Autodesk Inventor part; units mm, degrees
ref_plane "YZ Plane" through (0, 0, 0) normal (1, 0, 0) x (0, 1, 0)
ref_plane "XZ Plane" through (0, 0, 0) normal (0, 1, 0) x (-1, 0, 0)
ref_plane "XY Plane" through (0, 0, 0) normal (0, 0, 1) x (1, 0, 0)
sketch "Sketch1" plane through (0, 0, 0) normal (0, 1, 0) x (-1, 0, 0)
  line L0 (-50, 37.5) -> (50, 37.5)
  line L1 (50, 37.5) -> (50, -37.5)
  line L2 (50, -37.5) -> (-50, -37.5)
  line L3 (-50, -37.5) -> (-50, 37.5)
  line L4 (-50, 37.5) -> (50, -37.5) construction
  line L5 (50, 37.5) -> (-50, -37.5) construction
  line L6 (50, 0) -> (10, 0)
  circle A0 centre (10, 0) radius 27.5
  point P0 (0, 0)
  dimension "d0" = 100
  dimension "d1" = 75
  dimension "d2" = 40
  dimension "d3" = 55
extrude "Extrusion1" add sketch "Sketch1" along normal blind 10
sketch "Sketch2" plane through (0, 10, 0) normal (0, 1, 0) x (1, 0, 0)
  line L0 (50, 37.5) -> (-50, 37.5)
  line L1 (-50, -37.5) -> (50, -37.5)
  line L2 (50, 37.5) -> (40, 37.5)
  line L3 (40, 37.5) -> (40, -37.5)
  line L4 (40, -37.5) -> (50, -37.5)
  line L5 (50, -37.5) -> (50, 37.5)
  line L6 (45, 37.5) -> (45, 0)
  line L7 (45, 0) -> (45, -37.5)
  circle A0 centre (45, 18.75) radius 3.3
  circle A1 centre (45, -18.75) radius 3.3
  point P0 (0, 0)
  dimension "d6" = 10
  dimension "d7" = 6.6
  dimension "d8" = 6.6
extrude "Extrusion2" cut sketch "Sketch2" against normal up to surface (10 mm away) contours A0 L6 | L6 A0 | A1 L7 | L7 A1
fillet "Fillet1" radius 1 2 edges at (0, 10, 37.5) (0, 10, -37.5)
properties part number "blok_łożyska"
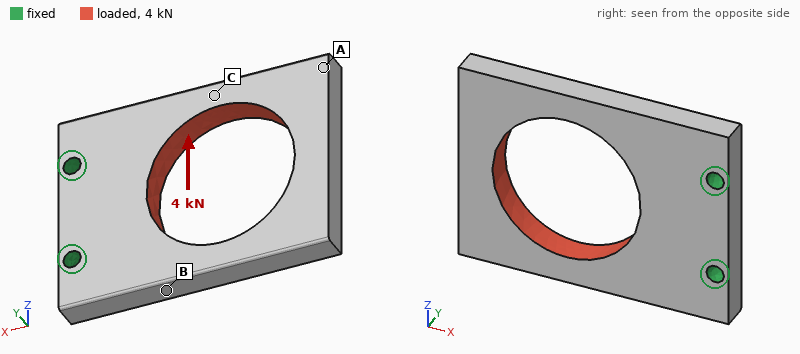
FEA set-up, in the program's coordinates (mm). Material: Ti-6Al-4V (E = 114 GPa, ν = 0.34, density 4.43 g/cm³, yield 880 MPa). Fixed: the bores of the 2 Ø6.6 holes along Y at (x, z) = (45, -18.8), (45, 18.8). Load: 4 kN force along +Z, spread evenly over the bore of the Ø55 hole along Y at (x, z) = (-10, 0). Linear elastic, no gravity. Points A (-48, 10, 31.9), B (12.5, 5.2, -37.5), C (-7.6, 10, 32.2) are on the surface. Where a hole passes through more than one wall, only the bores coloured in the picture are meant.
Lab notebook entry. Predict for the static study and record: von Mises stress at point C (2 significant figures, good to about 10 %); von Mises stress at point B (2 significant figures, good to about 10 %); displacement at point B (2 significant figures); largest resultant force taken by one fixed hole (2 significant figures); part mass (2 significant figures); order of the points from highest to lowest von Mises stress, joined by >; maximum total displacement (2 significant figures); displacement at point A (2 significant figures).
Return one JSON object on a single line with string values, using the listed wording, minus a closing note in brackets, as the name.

{"von Mises stress at point C": "31 MPa", "von Mises stress at point B": "53 MPa", "displacement at point B": "0.027 mm", "largest resultant force taken by one fixed hole": "5.3 kN", "part mass": "220 g", "order of the points from highest to lowest von Mises stress, joined by >": "B > C > A", "maximum total displacement": "0.11 mm", "displacement at point A": "0.10 mm"}
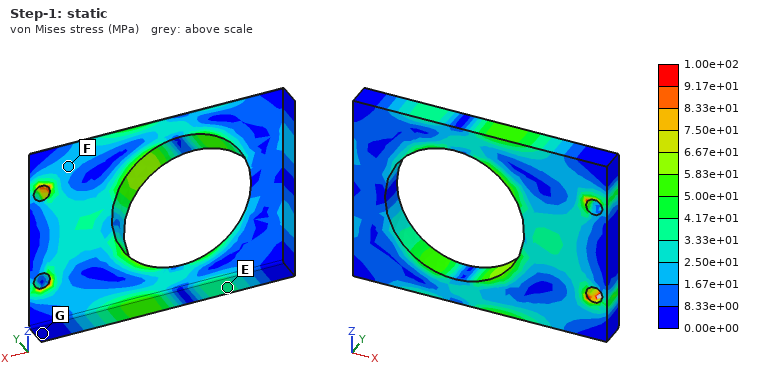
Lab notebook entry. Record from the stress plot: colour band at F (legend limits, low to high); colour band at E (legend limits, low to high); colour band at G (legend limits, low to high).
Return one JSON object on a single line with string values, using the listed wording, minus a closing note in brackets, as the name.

{"colour band at F": "1.67e+01 to 2.50e+01 MPa", "colour band at E": "3.33e+01 to 4.17e+01 MPa", "colour band at G": "0.00e+00 to 8.33e+00 MPa"}
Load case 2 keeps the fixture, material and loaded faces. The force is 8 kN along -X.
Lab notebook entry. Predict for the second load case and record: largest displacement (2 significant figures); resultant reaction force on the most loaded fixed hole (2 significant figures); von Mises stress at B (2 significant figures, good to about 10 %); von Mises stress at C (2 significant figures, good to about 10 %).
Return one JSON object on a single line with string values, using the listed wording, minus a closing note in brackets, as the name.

{"largest displacement": "35 µm", "resultant reaction force on the most loaded fixed hole": "4.2 kN", "von Mises stress at B": "30 MPa", "von Mises stress at C": "23 MPa"}
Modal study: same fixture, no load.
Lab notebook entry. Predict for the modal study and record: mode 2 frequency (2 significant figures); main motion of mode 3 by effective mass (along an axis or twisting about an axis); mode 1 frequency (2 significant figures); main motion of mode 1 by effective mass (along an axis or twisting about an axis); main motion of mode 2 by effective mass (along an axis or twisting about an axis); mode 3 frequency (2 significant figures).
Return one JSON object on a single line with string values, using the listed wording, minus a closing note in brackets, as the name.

{"mode 2 frequency": "1900 Hz", "main motion of mode 3 by effective mass": "along Z", "mode 1 frequency": "820 Hz", "main motion of mode 1 by effective mass": "along Y", "main motion of mode 2 by effective mass": "twisting about X", "mode 3 frequency": "2700 Hz"}
